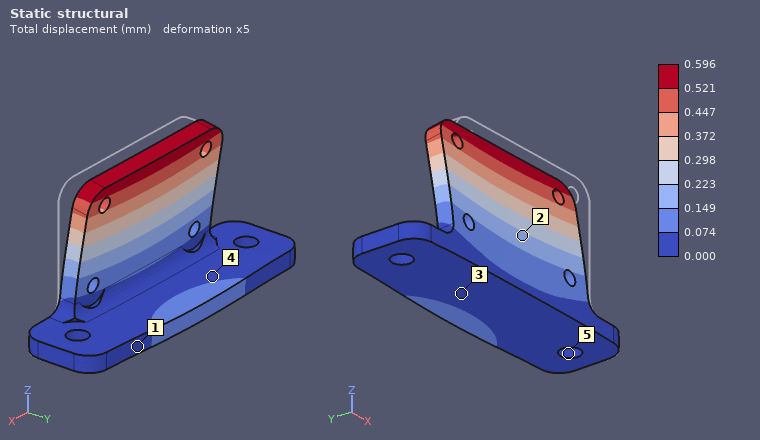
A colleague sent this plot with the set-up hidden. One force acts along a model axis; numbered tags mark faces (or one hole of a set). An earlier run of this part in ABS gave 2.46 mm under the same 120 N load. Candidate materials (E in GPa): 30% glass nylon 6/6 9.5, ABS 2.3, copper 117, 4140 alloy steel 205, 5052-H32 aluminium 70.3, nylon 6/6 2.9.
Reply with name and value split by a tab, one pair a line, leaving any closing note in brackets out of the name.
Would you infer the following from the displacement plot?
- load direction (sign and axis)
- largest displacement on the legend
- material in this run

load direction	+Y
largest displacement on the legend	0.596 mm
material in this run	30% glass nylon 6/6
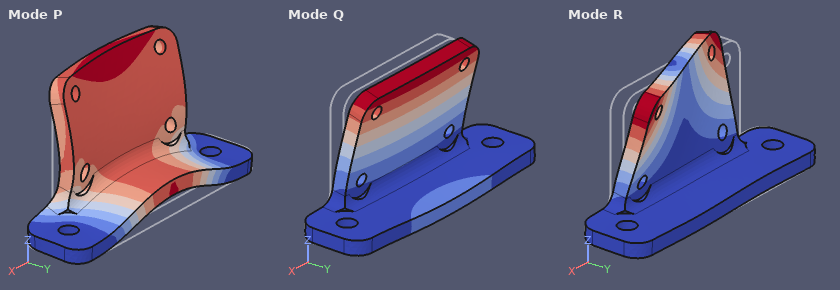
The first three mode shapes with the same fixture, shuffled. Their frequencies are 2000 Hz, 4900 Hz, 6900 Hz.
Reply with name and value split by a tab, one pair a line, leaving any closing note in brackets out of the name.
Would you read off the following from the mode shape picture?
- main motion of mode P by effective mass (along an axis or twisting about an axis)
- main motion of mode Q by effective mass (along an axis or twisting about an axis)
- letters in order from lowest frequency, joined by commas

main motion of mode P by effective mass	along Z
main motion of mode Q by effective mass	along Y
letters in order from lowest frequency, joined by commas	Q, R, P
